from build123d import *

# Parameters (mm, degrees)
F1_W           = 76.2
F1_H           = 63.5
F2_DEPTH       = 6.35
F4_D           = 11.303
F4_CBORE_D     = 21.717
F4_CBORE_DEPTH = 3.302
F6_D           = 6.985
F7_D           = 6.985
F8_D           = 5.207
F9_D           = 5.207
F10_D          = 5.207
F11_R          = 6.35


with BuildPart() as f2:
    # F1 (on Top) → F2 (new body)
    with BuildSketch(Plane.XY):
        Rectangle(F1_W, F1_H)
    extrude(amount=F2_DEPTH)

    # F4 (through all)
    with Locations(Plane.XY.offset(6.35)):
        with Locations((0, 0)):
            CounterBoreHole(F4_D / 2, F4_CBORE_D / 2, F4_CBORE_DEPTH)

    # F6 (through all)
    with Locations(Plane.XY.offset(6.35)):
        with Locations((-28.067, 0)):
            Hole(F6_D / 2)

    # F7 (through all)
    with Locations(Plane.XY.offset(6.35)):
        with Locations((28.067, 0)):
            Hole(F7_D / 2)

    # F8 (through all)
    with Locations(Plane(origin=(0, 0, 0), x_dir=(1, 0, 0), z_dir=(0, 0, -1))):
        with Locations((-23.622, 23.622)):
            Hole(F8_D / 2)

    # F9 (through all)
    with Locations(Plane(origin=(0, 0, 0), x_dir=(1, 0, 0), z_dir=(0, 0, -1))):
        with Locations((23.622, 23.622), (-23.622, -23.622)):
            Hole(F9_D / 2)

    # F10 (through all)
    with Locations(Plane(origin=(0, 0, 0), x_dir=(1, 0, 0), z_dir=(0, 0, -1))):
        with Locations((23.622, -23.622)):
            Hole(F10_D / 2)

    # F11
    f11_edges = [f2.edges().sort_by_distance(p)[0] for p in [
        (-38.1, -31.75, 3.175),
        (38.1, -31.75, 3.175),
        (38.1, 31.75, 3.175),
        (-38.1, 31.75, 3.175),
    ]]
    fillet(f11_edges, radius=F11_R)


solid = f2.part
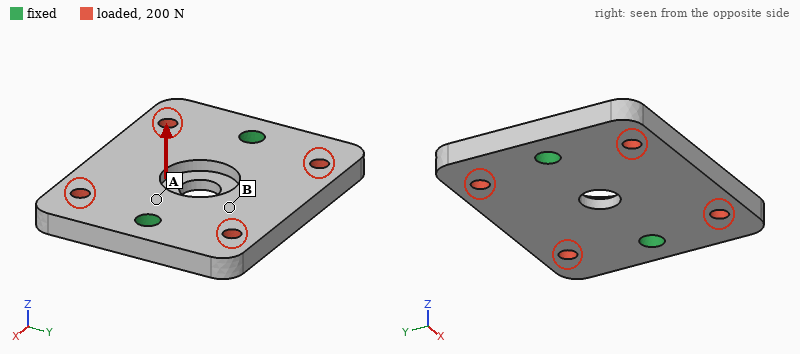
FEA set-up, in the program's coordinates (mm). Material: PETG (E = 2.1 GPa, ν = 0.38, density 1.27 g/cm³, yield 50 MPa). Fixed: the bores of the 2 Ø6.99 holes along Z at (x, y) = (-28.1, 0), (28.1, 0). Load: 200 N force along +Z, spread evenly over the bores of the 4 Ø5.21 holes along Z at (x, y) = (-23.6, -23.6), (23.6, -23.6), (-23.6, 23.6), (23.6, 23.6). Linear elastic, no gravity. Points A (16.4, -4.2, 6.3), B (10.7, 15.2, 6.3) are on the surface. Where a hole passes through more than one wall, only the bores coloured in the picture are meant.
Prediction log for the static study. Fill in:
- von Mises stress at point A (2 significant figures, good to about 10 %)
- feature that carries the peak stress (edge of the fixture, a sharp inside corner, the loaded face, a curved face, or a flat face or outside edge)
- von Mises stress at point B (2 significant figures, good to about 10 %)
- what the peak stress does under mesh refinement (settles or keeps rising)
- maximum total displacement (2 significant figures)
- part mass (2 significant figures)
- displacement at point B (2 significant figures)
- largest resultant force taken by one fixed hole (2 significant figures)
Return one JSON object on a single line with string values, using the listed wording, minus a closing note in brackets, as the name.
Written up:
{"von Mises stress at point A": "4.0 MPa", "feature that carries the peak stress": "edge of the fixture", "von Mises stress at point B": "1.3 MPa", "what the peak stress does under mesh refinement": "keeps rising", "maximum total displacement": "0.21 mm", "part mass": "35 g", "displacement at point B": "0.080 mm", "largest resultant force taken by one fixed hole": "100 N"}
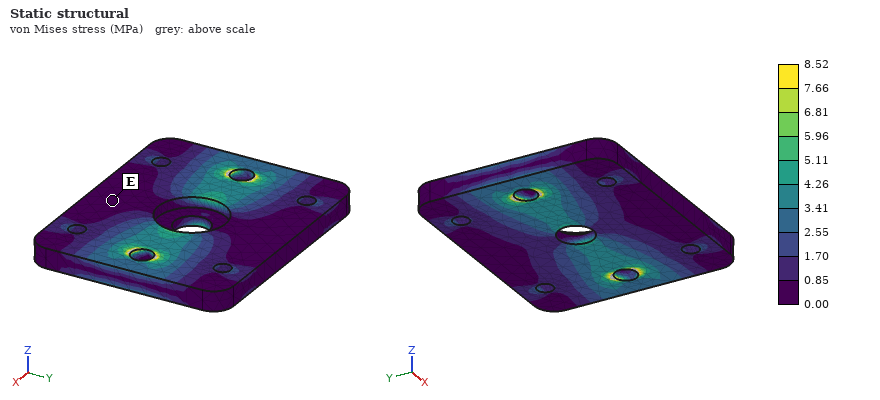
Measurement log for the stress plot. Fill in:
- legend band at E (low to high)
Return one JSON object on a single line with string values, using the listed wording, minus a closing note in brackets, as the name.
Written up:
{"legend band at E": "0.00 to 0.85 MPa"}
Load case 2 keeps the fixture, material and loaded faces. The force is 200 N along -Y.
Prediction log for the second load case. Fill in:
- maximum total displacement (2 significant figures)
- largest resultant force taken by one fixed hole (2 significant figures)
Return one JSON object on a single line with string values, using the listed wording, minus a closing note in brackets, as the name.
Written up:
{"maximum total displacement": "7.1 µm", "largest resultant force taken by one fixed hole": "100 N"}
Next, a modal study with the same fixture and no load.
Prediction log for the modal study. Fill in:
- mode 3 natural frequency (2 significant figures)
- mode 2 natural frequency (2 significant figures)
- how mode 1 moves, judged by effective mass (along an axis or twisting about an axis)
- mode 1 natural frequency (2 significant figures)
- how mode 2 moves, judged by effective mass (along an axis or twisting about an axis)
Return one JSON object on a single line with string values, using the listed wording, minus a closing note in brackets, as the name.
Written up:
{"mode 3 natural frequency": "1800 Hz", "mode 2 natural frequency": "1200 Hz", "how mode 1 moves, judged by effective mass": "twisting about X", "mode 1 natural frequency": "1000 Hz", "how mode 2 moves, judged by effective mass": "along Z"}
